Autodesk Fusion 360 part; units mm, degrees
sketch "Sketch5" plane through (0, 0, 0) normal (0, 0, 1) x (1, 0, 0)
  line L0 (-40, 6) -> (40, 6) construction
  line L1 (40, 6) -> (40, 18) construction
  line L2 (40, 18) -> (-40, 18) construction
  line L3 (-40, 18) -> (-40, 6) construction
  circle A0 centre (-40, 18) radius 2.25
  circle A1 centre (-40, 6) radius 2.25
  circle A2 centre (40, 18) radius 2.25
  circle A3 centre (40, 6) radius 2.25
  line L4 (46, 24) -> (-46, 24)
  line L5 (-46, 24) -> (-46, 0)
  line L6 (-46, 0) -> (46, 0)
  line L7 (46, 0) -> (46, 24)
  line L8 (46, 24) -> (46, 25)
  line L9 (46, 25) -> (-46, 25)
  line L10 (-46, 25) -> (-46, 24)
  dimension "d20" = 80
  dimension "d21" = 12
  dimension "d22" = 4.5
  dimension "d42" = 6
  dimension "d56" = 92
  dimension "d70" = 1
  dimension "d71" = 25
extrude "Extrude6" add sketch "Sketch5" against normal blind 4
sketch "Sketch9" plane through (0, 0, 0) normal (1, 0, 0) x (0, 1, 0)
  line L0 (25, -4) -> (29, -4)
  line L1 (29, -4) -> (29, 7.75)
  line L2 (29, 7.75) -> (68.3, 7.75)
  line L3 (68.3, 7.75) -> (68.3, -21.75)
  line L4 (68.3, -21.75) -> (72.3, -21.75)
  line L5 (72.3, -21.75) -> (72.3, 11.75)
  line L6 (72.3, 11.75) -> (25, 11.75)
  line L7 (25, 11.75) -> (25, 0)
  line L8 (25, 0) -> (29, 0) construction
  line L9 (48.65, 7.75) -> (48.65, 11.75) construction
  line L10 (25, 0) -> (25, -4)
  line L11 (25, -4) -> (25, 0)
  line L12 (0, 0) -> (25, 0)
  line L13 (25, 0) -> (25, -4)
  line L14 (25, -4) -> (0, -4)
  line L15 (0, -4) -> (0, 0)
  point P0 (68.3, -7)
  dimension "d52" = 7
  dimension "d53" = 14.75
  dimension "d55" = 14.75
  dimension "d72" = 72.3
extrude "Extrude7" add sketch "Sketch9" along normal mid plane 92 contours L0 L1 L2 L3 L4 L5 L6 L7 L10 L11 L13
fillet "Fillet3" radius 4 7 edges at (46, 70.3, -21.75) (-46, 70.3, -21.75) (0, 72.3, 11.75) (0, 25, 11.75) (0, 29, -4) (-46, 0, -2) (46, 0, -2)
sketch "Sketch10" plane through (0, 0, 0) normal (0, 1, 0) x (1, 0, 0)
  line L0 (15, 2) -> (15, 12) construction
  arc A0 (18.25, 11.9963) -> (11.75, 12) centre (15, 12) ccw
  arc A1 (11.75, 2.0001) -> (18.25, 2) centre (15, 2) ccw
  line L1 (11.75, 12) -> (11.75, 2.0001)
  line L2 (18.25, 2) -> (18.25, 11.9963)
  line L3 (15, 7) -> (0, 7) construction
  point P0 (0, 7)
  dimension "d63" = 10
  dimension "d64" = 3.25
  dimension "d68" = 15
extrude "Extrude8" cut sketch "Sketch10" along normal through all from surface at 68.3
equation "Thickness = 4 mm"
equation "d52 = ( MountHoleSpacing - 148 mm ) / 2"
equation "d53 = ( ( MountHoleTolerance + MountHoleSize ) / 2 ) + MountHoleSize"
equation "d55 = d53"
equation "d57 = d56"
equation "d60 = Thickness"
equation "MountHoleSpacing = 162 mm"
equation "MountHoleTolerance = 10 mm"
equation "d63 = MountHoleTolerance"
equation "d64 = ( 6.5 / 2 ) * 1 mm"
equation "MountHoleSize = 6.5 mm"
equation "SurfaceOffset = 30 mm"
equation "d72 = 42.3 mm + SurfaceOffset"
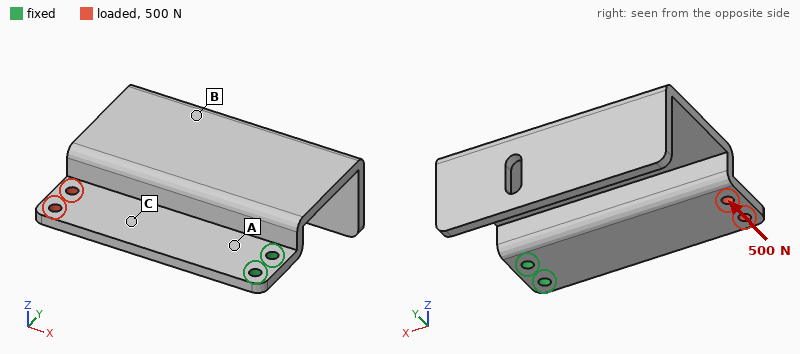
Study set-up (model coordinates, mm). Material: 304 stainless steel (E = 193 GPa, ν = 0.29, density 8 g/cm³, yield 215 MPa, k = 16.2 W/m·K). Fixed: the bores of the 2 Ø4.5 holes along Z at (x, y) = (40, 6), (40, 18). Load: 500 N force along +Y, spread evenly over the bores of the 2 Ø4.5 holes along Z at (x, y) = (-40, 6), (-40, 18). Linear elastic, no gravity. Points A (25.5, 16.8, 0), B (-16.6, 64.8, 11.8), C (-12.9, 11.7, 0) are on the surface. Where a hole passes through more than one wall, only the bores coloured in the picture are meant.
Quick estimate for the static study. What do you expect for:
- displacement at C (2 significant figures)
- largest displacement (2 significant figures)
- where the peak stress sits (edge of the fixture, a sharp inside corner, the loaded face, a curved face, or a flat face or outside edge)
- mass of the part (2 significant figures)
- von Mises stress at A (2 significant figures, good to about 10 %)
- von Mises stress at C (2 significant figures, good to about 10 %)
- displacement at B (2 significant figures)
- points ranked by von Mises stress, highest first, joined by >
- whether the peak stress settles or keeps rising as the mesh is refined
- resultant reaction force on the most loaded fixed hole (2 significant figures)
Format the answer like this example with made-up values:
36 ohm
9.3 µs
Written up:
44 µm
99 µm
edge of the fixture
320 g
19 MPa
11 MPa
60 µm
A > C > B
keeps rising
2.6 kN
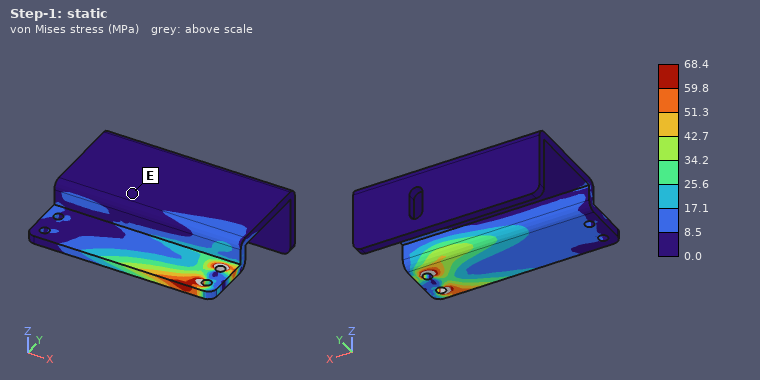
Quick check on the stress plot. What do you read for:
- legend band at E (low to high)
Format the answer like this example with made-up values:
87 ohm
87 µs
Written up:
0.0 to 8.5 MPa
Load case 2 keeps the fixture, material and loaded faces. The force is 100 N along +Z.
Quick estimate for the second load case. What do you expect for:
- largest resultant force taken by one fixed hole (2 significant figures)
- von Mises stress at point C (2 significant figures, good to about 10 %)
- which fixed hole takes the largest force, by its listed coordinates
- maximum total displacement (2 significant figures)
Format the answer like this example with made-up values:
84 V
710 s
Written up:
110 N
8.3 MPa
(40, 18)
0.16 mm
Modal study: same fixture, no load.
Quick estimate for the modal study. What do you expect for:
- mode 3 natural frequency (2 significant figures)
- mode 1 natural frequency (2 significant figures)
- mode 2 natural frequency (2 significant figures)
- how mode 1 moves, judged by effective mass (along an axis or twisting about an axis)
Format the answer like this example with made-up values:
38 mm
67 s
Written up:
850 Hz
270 Hz
610 Hz
along Z
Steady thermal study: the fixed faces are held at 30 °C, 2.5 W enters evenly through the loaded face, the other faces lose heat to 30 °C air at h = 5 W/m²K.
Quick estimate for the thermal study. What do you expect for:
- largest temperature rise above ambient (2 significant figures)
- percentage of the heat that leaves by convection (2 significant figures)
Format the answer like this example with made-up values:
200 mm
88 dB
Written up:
51 K
60 %
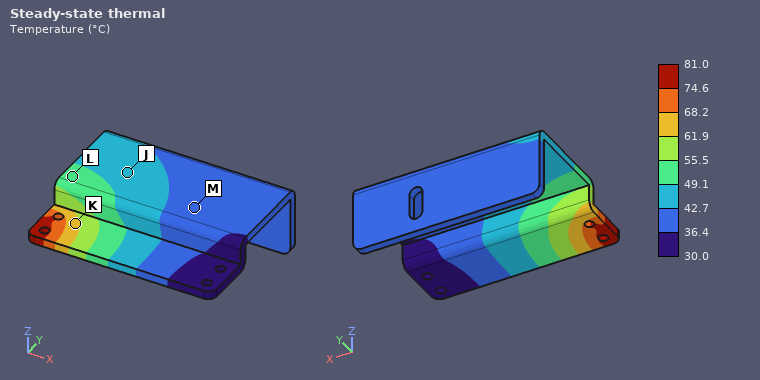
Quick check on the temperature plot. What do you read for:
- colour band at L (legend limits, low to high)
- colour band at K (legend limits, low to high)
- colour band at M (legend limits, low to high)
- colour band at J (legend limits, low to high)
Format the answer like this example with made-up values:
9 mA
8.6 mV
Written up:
49.1 to 55.5 °C
61.9 to 68.2 °C
36.4 to 42.7 °C
42.7 to 49.1 °C
